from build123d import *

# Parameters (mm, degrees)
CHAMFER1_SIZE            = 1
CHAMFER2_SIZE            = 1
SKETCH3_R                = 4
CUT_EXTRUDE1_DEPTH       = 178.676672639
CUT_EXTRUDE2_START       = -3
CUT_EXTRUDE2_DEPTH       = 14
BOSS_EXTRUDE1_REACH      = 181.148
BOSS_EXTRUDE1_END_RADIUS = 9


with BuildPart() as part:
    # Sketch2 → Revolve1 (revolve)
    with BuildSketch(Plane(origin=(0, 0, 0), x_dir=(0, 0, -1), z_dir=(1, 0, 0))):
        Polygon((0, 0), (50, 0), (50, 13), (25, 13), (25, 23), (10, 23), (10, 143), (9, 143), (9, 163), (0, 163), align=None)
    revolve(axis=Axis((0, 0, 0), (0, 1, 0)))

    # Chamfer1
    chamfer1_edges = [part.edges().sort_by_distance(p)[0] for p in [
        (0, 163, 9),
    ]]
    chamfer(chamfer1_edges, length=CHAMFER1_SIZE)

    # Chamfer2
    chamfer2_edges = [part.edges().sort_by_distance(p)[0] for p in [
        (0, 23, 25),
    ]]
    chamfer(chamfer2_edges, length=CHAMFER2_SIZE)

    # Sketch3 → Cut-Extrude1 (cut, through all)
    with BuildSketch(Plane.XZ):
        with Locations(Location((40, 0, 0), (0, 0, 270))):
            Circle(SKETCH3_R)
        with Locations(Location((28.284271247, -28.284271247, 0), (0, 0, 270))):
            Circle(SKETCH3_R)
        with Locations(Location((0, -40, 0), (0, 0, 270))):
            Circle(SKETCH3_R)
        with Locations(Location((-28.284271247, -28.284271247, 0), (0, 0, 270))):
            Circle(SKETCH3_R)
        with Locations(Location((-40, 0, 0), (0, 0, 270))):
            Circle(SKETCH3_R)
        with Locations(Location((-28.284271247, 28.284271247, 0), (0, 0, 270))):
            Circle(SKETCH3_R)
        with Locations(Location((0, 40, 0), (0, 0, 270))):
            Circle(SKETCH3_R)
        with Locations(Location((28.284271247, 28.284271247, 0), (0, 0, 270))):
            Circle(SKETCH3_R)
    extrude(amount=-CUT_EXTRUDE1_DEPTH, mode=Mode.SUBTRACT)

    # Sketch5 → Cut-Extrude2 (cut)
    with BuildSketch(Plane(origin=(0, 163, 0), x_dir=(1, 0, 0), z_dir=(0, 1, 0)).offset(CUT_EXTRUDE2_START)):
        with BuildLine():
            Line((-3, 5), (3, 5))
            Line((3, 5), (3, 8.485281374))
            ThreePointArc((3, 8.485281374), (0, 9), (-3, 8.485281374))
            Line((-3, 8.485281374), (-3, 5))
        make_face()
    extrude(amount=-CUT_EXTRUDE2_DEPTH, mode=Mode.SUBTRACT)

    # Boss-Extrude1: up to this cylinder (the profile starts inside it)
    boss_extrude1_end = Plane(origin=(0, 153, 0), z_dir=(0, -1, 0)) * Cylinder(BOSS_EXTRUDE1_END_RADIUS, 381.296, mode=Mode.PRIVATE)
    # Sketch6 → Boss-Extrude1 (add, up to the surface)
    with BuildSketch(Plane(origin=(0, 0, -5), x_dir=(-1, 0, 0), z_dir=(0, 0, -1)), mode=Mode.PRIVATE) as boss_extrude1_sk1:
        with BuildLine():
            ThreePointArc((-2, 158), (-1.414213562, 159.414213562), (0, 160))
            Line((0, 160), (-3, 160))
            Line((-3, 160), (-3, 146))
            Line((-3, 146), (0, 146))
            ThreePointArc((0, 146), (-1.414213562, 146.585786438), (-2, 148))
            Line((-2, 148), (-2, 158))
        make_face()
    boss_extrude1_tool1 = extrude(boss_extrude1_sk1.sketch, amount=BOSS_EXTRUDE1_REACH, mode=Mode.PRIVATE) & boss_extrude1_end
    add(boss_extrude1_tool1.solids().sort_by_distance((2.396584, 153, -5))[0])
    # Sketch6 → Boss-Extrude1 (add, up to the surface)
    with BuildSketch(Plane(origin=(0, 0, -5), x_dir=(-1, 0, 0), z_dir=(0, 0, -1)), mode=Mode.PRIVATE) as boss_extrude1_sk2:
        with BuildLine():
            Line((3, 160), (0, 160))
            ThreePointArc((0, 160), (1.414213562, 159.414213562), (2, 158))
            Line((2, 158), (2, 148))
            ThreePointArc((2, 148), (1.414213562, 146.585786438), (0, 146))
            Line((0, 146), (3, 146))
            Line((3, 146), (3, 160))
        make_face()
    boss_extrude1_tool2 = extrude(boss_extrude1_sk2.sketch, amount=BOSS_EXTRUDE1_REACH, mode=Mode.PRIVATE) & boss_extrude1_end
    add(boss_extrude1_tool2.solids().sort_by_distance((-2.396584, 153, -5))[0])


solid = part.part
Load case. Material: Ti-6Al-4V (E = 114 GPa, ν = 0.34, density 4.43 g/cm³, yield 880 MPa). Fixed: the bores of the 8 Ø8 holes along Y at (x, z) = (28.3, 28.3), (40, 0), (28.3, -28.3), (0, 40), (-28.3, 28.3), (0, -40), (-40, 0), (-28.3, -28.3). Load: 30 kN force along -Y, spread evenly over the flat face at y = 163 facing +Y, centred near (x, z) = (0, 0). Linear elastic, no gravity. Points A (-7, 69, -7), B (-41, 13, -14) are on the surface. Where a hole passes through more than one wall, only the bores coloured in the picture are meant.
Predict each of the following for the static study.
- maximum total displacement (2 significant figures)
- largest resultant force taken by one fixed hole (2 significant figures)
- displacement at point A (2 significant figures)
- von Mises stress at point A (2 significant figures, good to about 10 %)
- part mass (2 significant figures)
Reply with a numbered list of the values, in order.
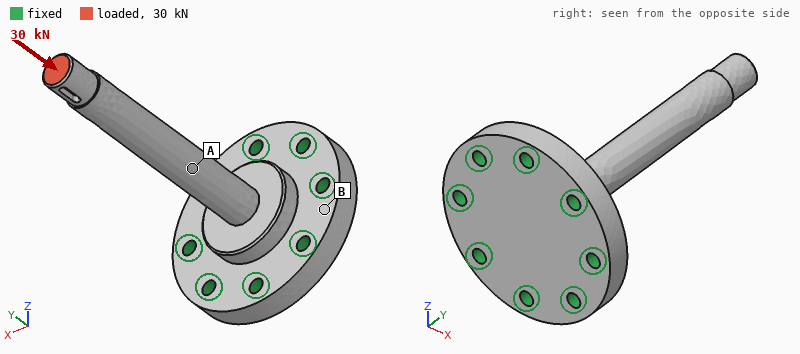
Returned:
1. 0.15 mm
2. 4.4 kN
3. 0.059 mm
4. 95 MPa
5. 700 g
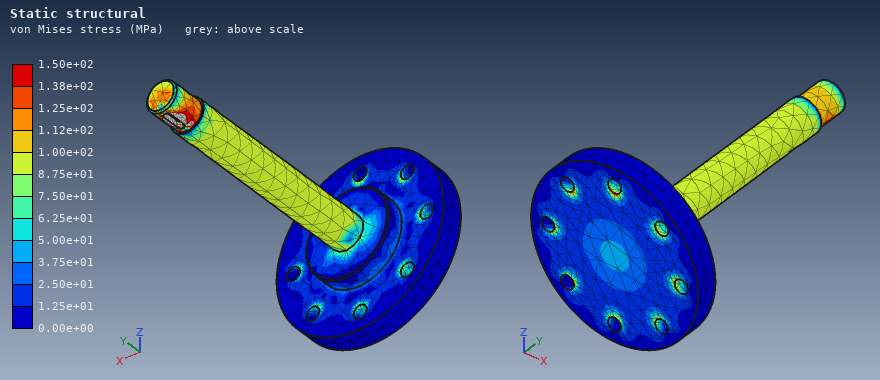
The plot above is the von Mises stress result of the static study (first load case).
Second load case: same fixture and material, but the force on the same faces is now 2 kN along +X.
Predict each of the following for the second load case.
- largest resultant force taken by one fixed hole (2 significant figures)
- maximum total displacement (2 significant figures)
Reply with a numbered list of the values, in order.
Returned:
1. 2.5 kN
2. 2.3 mm
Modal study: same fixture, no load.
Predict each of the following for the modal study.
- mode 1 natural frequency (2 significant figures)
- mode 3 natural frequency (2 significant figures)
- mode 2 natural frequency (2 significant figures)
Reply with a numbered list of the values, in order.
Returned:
1. 710 Hz
2. 4100 Hz
3. 710 Hz
